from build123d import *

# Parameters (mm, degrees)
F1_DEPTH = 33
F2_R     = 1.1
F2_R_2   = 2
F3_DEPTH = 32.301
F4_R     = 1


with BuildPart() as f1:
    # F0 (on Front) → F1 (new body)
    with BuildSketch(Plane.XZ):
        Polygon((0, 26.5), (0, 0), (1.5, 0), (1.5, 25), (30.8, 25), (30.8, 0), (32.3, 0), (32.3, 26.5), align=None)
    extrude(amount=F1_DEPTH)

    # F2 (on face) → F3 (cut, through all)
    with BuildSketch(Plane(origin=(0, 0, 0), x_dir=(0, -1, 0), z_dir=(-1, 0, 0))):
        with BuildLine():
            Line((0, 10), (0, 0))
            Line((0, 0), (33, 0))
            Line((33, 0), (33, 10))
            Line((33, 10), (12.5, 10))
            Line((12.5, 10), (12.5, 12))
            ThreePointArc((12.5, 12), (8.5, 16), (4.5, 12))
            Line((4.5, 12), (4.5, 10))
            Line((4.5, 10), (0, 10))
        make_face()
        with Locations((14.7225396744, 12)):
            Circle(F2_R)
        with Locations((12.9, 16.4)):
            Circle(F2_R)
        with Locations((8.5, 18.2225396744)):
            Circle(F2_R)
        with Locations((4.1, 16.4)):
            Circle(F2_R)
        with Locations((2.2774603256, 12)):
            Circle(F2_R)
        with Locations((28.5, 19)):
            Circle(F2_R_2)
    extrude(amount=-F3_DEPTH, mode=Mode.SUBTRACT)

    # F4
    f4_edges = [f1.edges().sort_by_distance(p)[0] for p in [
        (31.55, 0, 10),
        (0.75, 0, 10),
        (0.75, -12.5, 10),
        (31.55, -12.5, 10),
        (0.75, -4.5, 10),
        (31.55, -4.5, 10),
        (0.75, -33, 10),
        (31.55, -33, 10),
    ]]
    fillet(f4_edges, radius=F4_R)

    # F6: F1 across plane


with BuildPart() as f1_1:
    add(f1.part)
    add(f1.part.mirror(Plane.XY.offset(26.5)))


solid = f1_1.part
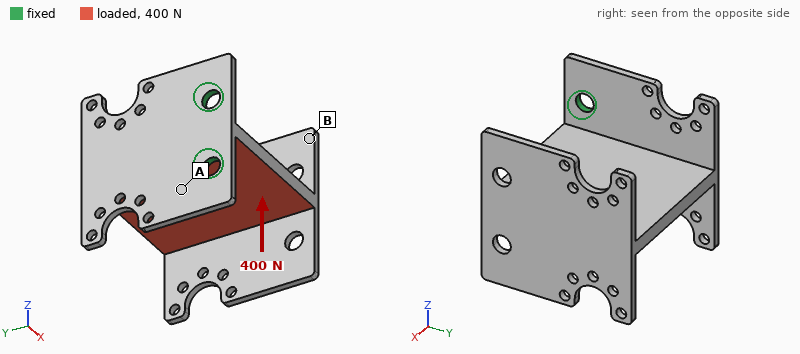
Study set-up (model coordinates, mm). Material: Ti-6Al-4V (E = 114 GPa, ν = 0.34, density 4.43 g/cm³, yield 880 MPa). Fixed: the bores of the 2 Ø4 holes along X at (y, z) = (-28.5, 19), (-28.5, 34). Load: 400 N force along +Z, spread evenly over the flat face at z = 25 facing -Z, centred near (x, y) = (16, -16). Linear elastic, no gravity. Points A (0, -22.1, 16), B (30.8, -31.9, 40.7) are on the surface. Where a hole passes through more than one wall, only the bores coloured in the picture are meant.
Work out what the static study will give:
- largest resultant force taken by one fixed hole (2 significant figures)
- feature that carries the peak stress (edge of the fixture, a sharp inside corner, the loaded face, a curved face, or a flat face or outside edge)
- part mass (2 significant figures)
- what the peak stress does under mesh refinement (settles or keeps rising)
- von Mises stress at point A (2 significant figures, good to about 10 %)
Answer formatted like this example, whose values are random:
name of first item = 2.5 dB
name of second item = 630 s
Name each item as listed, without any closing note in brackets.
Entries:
largest resultant force taken by one fixed hole = 670 N
feature that carries the peak stress = edge of the fixture
part mass = 25 g
what the peak stress does under mesh refinement = keeps rising
von Mises stress at point A = 45 MPa
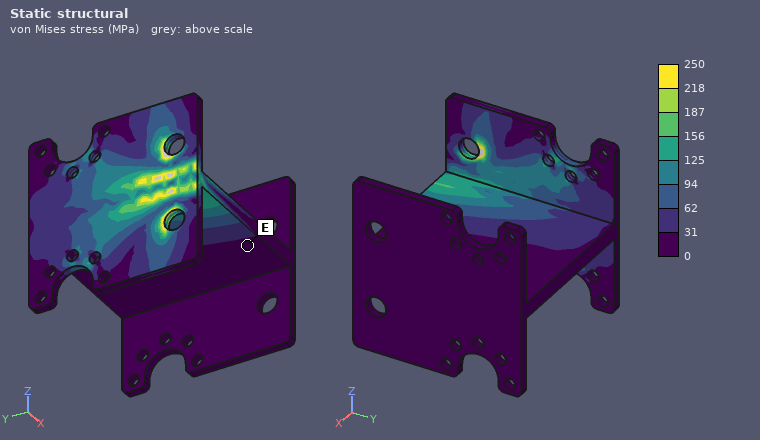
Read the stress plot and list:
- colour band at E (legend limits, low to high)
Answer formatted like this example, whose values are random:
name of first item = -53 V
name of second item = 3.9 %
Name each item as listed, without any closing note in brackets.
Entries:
colour band at E = 0 to 31 MPa
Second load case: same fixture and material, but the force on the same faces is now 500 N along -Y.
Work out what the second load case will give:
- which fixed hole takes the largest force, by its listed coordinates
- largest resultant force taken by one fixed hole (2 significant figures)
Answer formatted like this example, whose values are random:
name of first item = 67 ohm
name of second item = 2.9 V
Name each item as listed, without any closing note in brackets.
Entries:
which fixed hole takes the largest force, by its listed coordinates = (-28.5, 19)
largest resultant force taken by one fixed hole = 300 N
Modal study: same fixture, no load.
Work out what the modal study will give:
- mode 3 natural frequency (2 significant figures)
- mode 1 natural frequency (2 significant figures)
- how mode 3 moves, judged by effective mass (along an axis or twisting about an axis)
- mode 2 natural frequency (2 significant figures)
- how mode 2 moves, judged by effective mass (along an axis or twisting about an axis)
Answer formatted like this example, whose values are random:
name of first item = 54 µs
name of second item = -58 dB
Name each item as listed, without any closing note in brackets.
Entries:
mode 3 natural frequency = 2800 Hz
mode 1 natural frequency = 910 Hz
how mode 3 moves, judged by effective mass = twisting about X
mode 2 natural frequency = 950 Hz
how mode 2 moves, judged by effective mass = along Z
